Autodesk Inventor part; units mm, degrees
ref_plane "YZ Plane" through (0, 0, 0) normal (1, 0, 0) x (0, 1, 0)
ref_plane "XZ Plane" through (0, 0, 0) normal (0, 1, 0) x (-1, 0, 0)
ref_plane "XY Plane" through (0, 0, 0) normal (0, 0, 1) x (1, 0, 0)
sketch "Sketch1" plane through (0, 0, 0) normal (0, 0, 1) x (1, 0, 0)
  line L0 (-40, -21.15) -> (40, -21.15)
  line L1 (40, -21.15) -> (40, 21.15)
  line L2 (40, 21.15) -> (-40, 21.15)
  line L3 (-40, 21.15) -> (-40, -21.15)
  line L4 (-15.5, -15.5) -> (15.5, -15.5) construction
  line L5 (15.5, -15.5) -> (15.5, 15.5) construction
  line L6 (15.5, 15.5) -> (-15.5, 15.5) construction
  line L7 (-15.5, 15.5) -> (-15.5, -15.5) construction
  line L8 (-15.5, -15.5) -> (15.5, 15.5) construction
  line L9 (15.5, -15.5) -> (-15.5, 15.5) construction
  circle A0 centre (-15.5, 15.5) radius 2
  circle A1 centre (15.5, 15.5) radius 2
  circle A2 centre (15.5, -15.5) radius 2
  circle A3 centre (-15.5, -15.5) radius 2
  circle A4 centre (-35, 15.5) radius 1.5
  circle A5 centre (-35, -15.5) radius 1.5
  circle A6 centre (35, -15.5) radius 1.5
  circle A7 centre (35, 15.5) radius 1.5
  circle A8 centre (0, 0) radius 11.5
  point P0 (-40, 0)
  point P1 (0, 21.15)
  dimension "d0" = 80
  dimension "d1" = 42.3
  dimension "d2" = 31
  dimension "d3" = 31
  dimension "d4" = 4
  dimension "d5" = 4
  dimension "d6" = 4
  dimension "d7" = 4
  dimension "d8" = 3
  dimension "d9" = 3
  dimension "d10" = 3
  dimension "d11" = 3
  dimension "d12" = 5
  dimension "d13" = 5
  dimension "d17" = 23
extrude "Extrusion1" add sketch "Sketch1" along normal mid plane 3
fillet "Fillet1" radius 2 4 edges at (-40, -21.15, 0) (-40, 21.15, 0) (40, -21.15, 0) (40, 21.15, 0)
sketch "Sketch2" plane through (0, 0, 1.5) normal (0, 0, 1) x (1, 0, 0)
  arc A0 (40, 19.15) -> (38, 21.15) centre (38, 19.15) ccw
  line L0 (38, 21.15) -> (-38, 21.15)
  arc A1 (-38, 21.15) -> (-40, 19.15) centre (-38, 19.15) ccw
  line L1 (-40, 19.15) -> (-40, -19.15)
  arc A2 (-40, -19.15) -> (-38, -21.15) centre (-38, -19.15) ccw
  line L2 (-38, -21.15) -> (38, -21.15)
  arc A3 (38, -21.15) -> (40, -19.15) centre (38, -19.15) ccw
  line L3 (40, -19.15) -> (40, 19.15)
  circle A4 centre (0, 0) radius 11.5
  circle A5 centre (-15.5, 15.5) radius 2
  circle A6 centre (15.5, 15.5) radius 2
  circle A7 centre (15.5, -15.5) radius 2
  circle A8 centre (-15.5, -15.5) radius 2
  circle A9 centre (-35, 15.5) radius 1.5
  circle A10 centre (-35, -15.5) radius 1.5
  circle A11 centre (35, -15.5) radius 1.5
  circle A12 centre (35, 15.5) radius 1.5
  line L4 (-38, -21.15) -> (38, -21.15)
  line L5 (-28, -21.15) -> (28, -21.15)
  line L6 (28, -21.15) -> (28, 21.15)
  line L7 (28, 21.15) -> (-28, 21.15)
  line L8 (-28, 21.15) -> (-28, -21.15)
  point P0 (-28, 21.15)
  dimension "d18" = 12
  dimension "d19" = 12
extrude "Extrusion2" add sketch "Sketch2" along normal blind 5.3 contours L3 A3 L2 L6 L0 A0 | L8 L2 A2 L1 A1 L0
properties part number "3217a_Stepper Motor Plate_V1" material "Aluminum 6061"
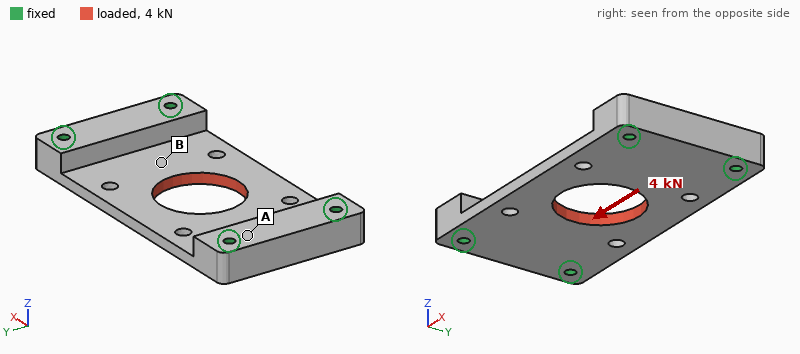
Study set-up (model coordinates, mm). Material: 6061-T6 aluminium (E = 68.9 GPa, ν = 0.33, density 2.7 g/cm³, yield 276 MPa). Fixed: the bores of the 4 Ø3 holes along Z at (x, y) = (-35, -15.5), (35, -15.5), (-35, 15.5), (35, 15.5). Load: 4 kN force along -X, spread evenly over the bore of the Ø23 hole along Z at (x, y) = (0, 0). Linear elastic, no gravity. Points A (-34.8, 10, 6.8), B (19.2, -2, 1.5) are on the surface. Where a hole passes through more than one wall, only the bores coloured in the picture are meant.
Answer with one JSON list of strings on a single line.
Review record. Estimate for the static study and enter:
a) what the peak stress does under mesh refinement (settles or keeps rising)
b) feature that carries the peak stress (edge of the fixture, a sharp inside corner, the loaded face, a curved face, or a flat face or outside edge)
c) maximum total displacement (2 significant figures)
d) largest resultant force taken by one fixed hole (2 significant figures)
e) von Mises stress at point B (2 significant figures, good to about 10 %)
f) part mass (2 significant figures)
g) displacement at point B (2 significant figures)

["keeps rising", "edge of the fixture", "11 µm", "1.0 kN", "18 MPa", "37 g", "7.5 µm"]
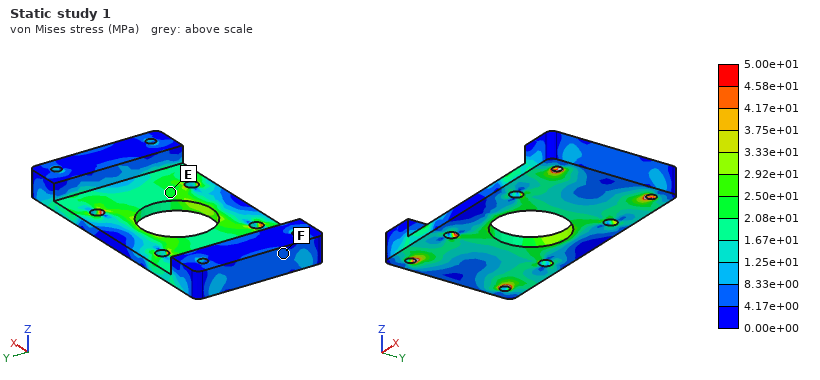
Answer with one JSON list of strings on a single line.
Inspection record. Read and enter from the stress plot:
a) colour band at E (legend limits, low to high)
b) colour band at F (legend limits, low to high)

["2.08e+01 to 2.50e+01 MPa", "4.17e+00 to 8.33e+00 MPa"]
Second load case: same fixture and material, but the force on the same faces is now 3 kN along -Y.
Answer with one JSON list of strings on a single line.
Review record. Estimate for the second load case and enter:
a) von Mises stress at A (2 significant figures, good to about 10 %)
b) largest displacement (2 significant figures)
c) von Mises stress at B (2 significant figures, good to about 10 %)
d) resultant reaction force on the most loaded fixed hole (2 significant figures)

["7.8 MPa", "21 µm", "35 MPa", "1.1 kN"]
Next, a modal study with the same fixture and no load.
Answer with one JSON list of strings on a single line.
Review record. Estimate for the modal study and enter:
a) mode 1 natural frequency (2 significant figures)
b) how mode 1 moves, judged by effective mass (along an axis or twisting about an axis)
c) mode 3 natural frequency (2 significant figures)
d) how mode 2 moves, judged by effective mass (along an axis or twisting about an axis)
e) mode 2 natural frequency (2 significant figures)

["4800 Hz", "along Z", "10 kHz", "twisting about X", "5700 Hz"]
